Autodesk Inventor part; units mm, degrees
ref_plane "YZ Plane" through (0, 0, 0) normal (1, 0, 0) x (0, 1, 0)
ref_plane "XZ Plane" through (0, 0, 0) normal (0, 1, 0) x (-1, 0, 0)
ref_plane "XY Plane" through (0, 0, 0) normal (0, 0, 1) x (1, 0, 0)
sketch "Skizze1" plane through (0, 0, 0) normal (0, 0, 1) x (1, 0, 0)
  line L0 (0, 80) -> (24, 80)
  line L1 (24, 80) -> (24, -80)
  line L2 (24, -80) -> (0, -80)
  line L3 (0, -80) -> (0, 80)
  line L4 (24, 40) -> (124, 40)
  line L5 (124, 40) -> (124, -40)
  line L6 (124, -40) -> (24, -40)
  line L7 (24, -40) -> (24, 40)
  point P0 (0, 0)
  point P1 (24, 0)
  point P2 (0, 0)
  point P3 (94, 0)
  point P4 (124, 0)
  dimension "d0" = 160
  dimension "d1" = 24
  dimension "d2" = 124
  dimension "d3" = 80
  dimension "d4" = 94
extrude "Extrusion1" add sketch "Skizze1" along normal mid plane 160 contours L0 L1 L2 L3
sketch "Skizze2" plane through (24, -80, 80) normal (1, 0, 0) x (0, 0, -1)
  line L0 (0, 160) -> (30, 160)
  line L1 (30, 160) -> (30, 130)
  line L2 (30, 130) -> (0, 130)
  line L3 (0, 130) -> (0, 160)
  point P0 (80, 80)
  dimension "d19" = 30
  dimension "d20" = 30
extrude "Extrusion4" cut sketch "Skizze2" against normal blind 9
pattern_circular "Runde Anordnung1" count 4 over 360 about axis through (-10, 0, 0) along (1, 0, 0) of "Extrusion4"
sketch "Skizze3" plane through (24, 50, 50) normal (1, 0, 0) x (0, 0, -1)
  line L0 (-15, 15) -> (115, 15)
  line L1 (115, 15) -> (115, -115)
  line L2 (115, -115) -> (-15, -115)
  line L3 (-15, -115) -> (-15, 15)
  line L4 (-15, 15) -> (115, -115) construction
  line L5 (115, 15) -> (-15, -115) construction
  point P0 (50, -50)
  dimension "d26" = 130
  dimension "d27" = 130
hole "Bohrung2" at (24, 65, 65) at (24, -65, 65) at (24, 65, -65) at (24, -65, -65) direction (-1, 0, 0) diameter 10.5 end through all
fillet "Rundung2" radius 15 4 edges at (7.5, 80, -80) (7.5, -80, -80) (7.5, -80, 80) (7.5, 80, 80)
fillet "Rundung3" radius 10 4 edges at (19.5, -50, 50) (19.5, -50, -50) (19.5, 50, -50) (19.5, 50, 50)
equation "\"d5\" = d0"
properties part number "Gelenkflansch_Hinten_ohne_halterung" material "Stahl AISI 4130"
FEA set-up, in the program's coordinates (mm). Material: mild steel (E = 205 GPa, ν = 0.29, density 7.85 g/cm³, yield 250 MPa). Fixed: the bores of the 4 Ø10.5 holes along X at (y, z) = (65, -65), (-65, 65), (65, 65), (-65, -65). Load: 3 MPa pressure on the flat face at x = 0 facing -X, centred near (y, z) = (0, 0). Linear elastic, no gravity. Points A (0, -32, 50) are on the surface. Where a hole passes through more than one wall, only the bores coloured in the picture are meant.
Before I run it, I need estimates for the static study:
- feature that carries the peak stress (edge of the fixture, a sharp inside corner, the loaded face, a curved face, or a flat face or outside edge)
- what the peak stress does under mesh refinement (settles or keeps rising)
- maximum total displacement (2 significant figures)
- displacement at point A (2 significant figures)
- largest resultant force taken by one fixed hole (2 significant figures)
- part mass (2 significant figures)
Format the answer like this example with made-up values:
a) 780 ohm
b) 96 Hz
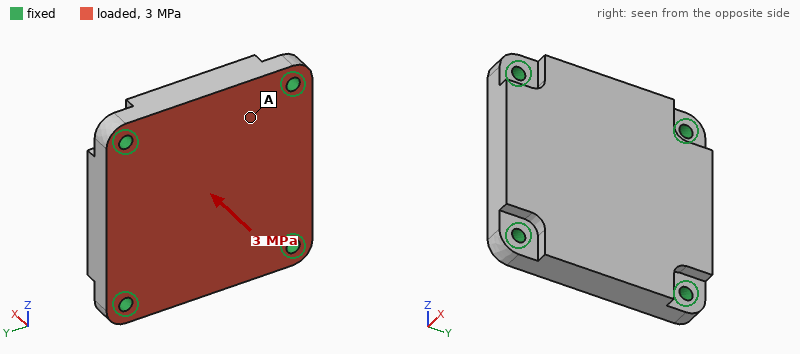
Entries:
a) edge of the fixture
b) keeps rising
c) 46 µm
d) 28 µm
e) 21 kN
f) 4.5 kg
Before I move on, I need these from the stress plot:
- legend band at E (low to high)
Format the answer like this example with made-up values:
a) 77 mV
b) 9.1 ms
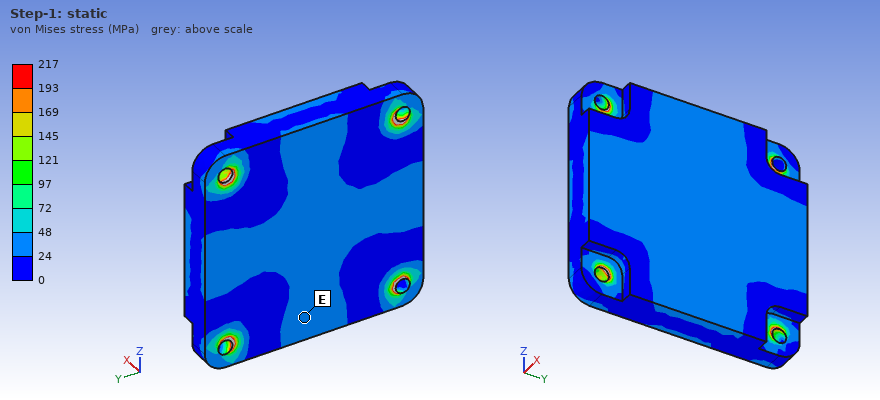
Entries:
a) 24 to 48 MPa
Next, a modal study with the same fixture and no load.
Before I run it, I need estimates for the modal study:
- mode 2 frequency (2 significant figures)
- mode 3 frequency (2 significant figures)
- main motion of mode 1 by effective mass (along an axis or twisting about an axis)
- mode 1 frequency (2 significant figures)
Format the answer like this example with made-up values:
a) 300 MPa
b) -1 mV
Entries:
a) 5600 Hz
b) 5600 Hz
c) along X
d) 3500 Hz
